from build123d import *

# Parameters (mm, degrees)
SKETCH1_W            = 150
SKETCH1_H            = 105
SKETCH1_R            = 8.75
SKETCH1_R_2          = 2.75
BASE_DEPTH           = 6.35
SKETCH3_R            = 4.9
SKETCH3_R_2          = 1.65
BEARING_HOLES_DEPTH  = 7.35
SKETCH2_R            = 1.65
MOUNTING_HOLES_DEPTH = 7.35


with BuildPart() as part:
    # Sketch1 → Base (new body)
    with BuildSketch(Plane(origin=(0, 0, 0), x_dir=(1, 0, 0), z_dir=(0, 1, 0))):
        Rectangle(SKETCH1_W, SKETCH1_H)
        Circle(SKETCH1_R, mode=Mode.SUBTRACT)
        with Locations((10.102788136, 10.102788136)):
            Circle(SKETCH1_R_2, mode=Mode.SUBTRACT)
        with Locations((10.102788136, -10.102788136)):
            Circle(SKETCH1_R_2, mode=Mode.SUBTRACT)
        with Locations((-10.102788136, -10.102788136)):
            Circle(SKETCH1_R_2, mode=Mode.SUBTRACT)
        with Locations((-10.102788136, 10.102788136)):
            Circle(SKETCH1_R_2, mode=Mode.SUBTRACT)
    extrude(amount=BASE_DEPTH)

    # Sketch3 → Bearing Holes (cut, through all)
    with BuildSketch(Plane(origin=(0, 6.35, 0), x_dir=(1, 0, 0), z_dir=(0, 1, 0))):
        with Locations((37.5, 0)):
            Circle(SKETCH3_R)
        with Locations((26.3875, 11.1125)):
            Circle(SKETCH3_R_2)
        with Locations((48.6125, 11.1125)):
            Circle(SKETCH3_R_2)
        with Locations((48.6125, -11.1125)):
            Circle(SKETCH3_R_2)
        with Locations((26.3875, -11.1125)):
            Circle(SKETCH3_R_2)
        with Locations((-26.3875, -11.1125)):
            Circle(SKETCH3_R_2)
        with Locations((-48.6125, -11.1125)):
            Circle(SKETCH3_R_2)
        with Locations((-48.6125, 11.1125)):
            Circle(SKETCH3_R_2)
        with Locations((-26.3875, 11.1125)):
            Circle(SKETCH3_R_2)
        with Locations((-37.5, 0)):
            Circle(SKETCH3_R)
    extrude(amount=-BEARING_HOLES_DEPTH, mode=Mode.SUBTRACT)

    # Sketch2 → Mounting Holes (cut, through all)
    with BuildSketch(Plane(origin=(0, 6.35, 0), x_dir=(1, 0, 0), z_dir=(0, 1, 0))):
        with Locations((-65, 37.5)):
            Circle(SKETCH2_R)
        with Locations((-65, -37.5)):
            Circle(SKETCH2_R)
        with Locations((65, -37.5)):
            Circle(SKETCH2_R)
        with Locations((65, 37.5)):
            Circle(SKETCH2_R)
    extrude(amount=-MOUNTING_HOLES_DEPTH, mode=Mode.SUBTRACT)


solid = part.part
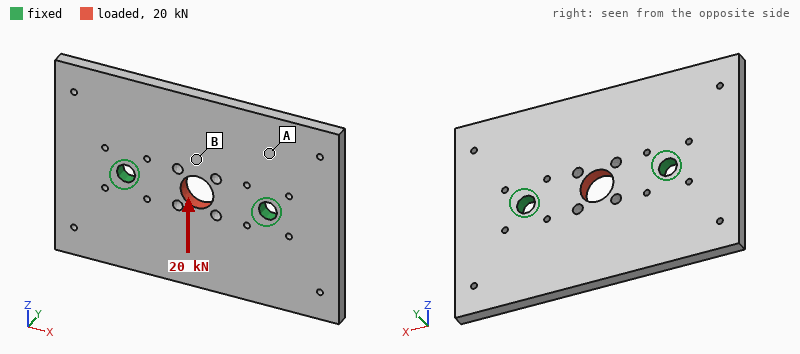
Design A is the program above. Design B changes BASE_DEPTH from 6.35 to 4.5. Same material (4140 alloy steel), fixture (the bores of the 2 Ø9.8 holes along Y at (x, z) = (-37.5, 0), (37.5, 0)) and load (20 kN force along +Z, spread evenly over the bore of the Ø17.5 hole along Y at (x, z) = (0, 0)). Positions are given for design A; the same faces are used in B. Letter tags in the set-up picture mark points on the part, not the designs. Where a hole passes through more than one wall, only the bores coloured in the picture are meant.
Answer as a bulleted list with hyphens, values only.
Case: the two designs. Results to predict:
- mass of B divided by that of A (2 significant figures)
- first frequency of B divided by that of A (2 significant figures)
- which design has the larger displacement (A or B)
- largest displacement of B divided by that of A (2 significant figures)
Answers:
- 0.71
- 0.74
- B
- 1.4
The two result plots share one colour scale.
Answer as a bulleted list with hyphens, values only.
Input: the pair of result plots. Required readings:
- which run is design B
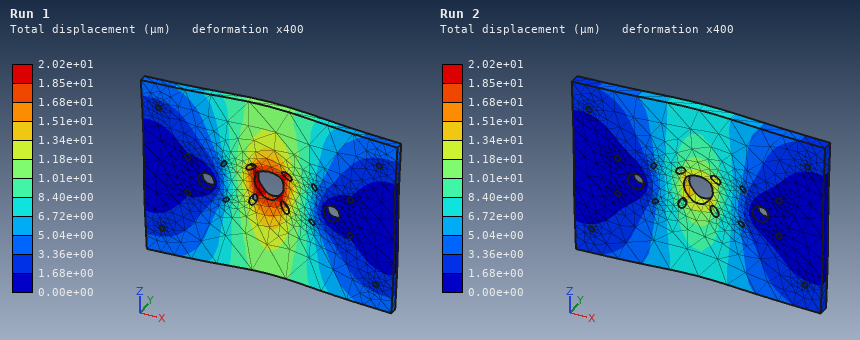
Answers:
- Run 1
